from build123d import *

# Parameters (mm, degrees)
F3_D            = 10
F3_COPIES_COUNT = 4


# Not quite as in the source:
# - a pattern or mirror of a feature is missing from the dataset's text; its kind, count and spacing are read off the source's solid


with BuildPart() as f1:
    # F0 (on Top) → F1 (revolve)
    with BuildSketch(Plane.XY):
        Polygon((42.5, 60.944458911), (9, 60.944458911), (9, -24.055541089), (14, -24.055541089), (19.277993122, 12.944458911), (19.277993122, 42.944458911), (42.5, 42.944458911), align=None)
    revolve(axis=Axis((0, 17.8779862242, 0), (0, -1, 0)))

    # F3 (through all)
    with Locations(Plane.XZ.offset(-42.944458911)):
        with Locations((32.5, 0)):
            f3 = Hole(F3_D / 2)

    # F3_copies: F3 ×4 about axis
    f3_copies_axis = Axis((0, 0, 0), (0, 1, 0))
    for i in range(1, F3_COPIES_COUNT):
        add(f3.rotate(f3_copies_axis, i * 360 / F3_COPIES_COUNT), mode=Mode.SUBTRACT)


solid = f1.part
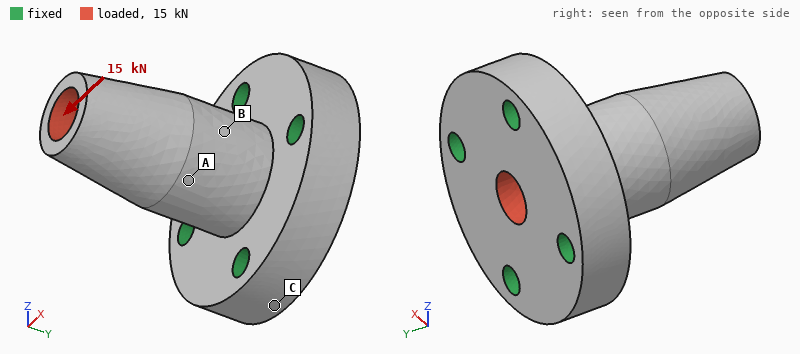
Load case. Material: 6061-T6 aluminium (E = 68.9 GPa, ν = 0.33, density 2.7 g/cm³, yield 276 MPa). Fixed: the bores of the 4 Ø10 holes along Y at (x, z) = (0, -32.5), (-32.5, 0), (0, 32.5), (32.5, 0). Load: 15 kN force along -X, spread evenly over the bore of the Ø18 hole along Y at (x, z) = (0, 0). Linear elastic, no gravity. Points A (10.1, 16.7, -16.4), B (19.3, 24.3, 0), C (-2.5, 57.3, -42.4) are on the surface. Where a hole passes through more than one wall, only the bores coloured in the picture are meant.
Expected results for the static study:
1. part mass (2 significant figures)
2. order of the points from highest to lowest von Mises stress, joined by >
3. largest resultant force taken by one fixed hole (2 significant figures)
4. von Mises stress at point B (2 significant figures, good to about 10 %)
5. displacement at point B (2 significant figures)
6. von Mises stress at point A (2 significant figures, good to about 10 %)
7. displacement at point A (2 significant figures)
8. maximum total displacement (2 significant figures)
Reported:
380 g
B > A > C
9.8 kN
36 MPa
0.050 mm
21 MPa
0.056 mm
0.15 mm
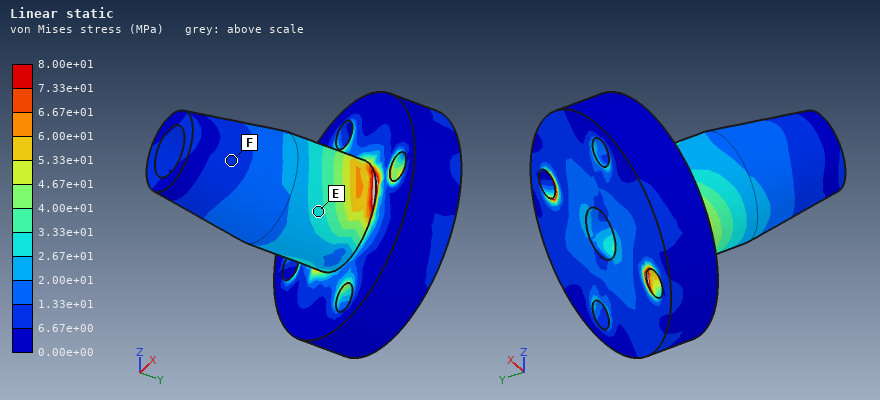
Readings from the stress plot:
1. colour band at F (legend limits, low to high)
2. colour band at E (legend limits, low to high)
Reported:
6.67e+00 to 1.33e+01 MPa
2.67e+01 to 3.33e+01 MPa
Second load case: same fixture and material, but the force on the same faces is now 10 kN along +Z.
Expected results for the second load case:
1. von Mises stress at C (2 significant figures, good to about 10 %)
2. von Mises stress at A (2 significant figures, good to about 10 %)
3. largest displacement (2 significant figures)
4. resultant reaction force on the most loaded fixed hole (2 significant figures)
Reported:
4.8 MPa
16 MPa
99 µm
6.5 kN
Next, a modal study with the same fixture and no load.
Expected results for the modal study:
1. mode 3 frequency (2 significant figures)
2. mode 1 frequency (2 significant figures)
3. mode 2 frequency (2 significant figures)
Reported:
13 kHz
5300 Hz
5300 Hz
